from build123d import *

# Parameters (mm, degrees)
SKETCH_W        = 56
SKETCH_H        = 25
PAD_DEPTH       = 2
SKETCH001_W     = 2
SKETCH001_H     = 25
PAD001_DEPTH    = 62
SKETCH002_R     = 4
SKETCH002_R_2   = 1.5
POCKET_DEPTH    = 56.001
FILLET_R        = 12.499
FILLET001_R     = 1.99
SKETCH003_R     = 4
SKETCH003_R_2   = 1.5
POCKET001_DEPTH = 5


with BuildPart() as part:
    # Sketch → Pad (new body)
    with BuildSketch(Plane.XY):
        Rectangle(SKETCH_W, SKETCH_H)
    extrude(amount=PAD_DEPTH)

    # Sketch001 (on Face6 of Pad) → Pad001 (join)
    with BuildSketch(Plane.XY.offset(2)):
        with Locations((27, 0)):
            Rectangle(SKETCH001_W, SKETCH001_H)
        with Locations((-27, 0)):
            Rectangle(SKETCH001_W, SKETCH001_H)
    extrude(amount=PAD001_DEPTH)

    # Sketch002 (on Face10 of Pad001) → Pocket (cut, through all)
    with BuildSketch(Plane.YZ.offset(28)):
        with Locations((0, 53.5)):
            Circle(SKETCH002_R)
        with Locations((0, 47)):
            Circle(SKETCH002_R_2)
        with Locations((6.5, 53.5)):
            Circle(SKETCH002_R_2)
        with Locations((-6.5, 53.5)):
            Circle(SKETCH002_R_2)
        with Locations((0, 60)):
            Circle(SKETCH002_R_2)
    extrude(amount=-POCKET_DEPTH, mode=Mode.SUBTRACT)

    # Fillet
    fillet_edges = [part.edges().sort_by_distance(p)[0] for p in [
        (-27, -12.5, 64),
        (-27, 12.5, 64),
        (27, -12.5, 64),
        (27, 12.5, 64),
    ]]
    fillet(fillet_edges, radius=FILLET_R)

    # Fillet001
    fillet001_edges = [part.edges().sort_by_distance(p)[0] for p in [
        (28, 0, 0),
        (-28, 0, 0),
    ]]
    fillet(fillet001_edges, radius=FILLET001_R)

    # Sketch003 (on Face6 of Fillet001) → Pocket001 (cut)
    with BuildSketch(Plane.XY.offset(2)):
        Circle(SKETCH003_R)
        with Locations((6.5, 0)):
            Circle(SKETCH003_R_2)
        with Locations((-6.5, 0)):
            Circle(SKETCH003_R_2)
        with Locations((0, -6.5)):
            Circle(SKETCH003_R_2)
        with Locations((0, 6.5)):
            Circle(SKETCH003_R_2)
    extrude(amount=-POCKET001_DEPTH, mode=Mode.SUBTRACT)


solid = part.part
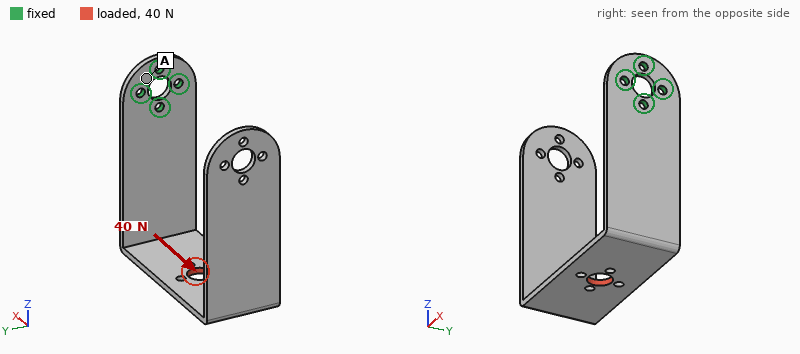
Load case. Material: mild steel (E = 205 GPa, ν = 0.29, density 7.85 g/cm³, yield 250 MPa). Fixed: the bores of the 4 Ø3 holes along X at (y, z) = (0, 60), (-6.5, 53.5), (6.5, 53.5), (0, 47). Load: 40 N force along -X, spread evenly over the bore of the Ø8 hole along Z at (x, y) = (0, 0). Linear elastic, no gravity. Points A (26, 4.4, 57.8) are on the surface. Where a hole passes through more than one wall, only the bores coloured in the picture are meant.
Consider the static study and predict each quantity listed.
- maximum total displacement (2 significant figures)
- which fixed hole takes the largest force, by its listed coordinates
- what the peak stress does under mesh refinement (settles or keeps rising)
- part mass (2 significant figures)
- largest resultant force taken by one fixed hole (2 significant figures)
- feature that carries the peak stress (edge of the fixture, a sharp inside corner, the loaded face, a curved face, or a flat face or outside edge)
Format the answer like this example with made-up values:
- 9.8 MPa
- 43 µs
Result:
- 0.77 mm
- (0, 47)
- keeps rising
- 65 g
- 170 N
- edge of the fixture
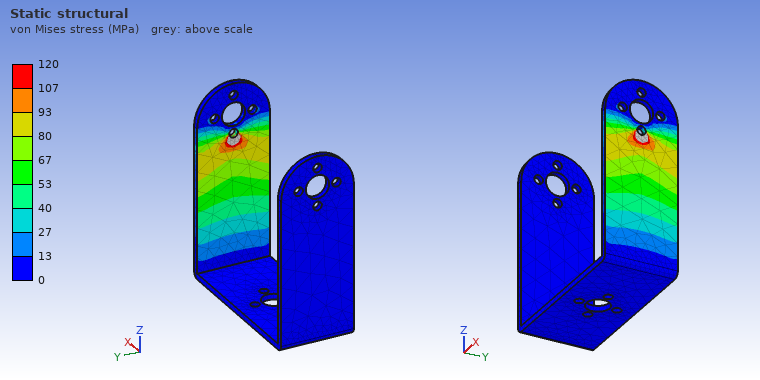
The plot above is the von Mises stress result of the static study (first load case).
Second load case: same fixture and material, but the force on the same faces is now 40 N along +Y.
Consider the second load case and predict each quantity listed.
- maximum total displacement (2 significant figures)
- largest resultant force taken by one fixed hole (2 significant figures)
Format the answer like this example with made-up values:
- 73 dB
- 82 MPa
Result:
- 0.54 mm
- 97 N
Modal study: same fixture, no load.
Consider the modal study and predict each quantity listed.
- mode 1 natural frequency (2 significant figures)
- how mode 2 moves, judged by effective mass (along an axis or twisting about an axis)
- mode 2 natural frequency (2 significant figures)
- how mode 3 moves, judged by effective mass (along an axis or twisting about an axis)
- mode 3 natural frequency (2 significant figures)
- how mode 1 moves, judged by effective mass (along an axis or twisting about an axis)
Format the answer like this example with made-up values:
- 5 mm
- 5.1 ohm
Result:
- 110 Hz
- along Y
- 160 Hz
- along X
- 250 Hz
- along Z
